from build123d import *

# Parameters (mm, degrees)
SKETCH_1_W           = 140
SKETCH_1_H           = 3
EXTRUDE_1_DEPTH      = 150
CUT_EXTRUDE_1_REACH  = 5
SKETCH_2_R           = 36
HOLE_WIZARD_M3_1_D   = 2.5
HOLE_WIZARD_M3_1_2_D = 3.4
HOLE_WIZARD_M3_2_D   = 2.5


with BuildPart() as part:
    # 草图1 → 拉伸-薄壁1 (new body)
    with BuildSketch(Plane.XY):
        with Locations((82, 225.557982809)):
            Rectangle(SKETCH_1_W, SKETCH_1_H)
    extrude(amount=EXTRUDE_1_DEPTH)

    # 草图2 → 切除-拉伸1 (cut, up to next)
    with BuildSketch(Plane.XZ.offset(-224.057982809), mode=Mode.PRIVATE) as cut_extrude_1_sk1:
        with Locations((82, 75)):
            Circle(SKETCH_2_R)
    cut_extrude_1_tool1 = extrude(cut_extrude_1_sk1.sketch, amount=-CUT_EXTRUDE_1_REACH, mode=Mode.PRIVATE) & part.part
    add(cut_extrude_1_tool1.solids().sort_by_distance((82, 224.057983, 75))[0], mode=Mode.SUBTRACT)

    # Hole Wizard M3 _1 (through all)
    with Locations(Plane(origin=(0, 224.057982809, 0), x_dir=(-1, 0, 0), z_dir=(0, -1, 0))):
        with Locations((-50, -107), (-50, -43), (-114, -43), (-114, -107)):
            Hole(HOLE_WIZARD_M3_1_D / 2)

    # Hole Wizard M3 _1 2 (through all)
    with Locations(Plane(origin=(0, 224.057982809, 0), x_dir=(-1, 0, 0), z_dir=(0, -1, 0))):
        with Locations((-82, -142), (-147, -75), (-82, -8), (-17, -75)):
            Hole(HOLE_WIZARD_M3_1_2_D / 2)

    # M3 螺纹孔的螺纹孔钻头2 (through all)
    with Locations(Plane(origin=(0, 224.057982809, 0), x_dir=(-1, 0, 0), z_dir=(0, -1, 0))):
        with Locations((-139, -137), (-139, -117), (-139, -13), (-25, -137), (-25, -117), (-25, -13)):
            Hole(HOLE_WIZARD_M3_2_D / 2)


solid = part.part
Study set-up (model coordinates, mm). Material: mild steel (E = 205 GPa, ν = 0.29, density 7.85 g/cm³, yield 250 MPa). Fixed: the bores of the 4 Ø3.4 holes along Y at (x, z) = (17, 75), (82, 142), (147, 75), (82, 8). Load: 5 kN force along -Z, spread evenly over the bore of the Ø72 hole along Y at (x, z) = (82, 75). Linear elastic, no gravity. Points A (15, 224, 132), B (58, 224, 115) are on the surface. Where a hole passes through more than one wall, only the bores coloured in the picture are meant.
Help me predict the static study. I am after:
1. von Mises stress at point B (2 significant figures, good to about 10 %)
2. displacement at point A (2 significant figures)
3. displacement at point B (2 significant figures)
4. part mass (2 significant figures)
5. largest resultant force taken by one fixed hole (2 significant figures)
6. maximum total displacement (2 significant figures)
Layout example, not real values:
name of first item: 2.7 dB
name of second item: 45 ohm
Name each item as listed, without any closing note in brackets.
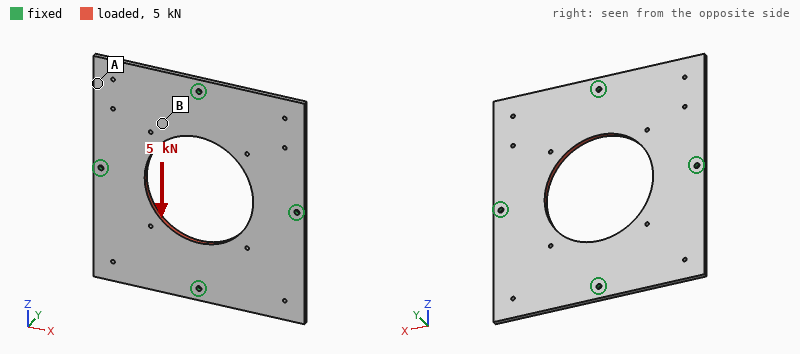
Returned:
von Mises stress at point B: 9.0 MPa
displacement at point A: 2.7 µm
displacement at point B: 3.1 µm
part mass: 400 g
largest resultant force taken by one fixed hole: 1.3 kN
maximum total displacement: 4.1 µm
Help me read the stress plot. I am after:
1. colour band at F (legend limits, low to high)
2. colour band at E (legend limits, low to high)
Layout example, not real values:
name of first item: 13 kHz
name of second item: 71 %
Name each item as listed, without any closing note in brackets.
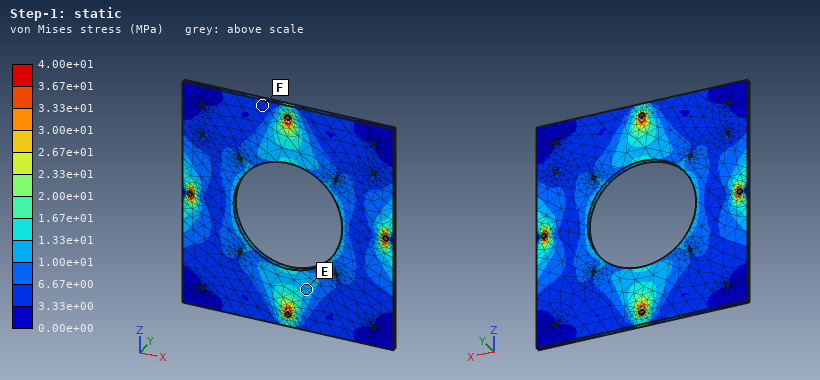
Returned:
colour band at F: 3.33e+00 to 6.67e+00 MPa
colour band at E: 1.00e+01 to 1.33e+01 MPa
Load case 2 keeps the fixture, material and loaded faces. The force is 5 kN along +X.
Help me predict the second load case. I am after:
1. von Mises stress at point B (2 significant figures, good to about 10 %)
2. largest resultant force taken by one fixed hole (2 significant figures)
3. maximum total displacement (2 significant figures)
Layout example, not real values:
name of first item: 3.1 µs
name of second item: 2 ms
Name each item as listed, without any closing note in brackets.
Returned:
von Mises stress at point B: 7.0 MPa
largest resultant force taken by one fixed hole: 1.3 kN
maximum total displacement: 4.1 µm
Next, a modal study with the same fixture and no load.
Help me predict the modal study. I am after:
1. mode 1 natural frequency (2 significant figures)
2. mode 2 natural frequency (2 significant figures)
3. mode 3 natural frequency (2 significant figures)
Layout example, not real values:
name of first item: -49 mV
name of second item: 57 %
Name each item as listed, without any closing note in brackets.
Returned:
mode 1 natural frequency: 820 Hz
mode 2 natural frequency: 870 Hz
mode 3 natural frequency: 890 Hz
